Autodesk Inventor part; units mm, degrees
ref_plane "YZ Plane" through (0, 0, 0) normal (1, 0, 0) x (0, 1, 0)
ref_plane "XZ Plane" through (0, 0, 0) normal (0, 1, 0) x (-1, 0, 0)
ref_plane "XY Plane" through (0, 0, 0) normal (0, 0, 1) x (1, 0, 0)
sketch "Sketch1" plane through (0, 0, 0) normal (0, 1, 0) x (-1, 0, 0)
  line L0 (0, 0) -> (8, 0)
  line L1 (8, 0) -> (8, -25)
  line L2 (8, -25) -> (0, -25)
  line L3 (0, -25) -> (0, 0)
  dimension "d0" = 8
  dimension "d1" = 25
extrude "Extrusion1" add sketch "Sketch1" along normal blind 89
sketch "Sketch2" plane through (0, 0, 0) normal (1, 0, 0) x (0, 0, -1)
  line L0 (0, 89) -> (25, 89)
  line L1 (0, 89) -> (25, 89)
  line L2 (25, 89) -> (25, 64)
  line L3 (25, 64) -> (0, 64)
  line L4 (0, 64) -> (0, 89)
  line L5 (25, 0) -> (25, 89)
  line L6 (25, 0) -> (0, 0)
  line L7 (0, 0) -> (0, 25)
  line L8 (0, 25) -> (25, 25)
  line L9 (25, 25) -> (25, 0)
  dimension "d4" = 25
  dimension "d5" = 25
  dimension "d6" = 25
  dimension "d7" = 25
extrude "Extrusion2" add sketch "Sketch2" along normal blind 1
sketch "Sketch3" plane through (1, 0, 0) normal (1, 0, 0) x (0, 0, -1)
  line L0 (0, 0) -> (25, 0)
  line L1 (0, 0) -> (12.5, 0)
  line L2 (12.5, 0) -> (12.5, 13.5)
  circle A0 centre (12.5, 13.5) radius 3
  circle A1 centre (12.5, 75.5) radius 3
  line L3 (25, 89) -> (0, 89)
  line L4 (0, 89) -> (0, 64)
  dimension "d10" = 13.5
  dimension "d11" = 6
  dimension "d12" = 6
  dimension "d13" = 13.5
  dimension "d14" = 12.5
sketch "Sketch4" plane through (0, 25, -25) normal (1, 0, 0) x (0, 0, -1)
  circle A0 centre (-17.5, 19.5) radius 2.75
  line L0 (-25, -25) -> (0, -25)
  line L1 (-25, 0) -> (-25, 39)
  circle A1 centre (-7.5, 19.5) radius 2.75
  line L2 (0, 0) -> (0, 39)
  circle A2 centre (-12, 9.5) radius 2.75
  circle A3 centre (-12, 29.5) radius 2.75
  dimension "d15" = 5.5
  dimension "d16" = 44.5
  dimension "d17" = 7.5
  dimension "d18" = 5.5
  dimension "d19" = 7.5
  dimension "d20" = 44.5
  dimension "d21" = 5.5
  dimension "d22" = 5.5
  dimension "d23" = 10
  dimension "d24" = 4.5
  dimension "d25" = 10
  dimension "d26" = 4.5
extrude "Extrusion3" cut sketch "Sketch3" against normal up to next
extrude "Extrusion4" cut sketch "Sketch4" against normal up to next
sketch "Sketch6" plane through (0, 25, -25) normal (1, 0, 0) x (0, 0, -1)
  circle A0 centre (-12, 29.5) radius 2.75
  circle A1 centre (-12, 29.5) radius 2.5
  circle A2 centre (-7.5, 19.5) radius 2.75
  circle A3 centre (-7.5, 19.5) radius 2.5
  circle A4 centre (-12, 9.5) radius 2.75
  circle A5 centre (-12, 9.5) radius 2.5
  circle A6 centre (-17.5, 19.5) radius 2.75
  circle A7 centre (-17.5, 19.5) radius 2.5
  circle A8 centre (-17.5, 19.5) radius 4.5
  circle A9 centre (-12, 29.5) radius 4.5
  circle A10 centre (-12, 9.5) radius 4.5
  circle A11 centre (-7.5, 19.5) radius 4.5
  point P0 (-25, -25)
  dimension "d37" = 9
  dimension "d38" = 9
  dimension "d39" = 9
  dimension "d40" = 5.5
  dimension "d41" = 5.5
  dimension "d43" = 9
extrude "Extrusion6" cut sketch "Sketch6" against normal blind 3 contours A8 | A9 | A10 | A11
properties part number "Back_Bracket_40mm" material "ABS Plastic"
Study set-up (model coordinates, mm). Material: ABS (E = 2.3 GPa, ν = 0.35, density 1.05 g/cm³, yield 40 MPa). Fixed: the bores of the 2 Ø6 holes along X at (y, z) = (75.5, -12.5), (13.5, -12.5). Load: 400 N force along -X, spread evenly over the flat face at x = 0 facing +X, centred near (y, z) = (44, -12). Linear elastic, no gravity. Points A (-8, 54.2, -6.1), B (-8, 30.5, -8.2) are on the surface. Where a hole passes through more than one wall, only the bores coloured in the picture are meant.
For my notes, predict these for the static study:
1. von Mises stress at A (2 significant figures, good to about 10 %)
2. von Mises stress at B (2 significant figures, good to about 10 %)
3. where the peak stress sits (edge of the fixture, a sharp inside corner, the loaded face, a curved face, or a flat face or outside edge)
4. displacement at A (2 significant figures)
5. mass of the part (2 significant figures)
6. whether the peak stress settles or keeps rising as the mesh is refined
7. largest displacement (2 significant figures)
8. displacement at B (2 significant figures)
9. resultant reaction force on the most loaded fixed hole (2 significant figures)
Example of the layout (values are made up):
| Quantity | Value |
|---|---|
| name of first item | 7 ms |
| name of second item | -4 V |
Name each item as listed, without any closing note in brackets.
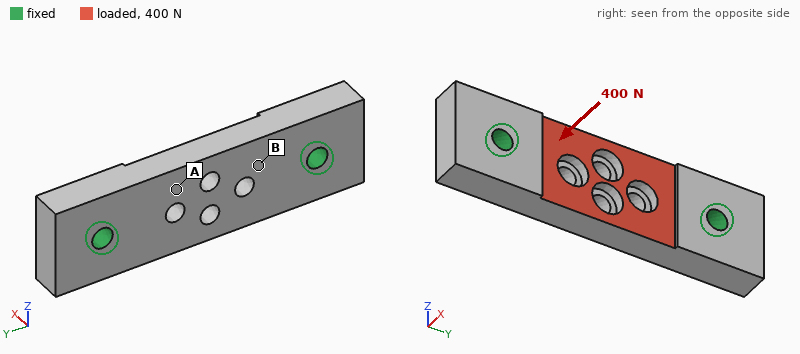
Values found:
| Quantity | Value |
|---|---|
| von Mises stress at A | 2.9 MPa |
| von Mises stress at B | 1.4 MPa |
| where the peak stress sits | edge of the fixture |
| displacement at A | 0.13 mm |
| mass of the part | 18 g |
| whether the peak stress settles or keeps rising as the mesh is refined | keeps rising |
| largest displacement | 0.18 mm |
| displacement at B | 0.10 mm |
| resultant reaction force on the most loaded fixed hole | 210 N |
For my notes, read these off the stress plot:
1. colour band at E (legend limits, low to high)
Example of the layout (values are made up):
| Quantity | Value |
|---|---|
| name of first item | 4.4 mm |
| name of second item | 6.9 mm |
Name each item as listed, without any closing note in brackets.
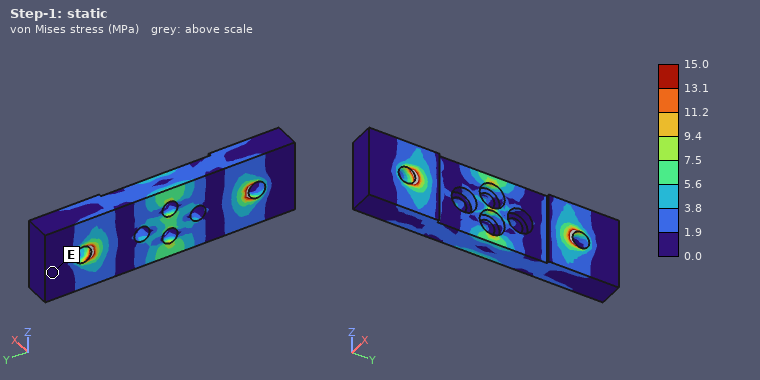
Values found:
| Quantity | Value |
|---|---|
| colour band at E | 0.0 to 1.9 MPa |
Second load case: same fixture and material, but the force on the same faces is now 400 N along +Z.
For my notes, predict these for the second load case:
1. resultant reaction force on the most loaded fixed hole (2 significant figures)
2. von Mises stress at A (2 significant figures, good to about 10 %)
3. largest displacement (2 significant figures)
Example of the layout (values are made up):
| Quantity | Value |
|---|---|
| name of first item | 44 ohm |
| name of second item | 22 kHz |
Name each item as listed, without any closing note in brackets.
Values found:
| Quantity | Value |
|---|---|
| resultant reaction force on the most loaded fixed hole | 200 N |
| von Mises stress at A | 1.4 MPa |
| largest displacement | 0.10 mm |
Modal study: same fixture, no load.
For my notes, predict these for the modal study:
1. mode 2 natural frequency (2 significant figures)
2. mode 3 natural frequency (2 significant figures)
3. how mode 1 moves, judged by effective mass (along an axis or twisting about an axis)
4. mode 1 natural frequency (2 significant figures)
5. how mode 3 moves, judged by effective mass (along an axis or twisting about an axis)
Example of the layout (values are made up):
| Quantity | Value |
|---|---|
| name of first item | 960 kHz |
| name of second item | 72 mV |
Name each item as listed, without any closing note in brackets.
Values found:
| Quantity | Value |
|---|---|
| mode 2 natural frequency | 4400 Hz |
| mode 3 natural frequency | 4700 Hz |
| how mode 1 moves, judged by effective mass | along X |
| mode 1 natural frequency | 3200 Hz |
| how mode 3 moves, judged by effective mass | along Z |
